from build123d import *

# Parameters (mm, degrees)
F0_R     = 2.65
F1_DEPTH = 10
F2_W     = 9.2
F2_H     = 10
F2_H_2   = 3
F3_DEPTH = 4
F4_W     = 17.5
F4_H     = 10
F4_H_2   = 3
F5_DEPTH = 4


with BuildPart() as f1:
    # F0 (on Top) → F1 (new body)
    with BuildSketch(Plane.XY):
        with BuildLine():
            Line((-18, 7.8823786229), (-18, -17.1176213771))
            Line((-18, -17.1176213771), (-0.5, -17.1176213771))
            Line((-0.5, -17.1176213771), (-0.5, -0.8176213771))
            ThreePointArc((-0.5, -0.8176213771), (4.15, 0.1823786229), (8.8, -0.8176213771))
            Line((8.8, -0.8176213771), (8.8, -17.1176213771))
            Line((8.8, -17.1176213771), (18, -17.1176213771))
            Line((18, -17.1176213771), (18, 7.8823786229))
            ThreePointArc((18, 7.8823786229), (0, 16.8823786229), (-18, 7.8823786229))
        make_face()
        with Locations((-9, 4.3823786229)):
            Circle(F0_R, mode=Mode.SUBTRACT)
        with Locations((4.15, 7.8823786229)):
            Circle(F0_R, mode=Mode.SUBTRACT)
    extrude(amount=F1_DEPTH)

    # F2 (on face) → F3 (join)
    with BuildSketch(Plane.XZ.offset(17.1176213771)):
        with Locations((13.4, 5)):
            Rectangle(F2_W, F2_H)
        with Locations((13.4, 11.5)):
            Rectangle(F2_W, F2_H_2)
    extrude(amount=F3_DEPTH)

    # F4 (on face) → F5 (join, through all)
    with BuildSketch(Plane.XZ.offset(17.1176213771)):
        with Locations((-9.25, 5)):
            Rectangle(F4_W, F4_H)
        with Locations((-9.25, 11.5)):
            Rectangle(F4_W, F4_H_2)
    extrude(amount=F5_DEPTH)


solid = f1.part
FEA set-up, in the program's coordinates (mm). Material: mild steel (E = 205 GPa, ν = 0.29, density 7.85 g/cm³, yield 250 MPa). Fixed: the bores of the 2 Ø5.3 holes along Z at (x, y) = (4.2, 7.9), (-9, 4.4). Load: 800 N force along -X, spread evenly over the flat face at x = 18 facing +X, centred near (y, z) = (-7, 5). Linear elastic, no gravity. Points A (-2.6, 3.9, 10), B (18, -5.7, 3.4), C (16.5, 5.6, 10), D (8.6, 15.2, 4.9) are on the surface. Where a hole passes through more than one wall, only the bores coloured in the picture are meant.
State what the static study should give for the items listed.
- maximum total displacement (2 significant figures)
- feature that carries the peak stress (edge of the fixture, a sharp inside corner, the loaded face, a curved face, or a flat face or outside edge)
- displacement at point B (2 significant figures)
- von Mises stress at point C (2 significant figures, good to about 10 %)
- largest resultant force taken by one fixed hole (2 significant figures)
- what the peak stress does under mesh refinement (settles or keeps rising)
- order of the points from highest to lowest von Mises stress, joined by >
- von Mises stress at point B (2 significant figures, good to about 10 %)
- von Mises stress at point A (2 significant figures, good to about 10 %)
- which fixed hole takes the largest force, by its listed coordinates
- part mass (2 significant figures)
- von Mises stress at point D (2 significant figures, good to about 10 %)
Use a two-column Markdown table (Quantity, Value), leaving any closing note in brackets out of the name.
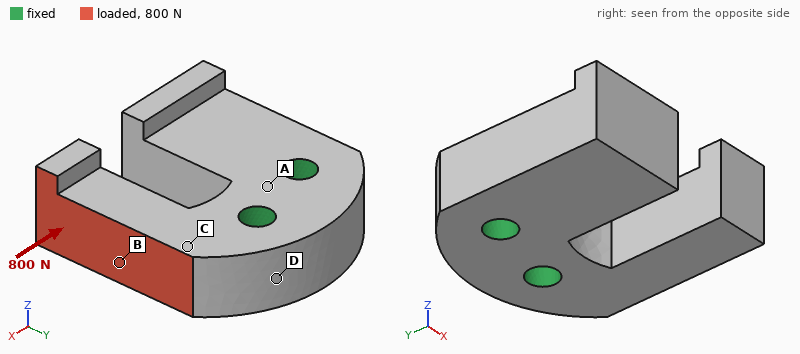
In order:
| Quantity | Value |
|---|---|
| maximum total displacement | 18 µm |
| feature that carries the peak stress | a sharp inside corner |
| displacement at point B | 7.2 µm |
| von Mises stress at point C | 21 MPa |
| largest resultant force taken by one fixed hole | 610 N |
| what the peak stress does under mesh refinement | keeps rising |
| order of the points from highest to lowest von Mises stress, joined by > | B > C > D > A |
| von Mises stress at point B | 27 MPa |
| von Mises stress at point A | 8.5 MPa |
| which fixed hole takes the largest force, by its listed coordinates | (4.2, 7.9) |
| part mass | 83 g |
| von Mises stress at point D | 16 MPa |
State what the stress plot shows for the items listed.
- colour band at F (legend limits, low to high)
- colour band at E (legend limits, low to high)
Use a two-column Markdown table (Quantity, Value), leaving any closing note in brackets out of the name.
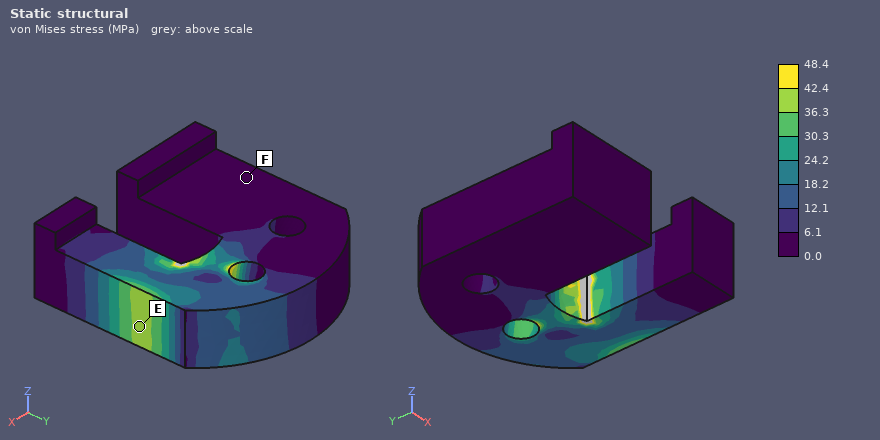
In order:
| Quantity | Value |
|---|---|
| colour band at F | 0.0 to 6.1 MPa |
| colour band at E | 36.3 to 42.4 MPa |
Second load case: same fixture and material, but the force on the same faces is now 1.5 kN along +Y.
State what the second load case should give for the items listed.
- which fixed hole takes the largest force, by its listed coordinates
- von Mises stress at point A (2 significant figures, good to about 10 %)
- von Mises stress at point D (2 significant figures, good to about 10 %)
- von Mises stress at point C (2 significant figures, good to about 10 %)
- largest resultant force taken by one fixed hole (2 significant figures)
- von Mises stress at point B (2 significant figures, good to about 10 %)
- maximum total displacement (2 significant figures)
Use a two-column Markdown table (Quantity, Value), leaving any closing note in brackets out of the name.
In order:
| Quantity | Value |
|---|---|
| which fixed hole takes the largest force, by its listed coordinates | (4.2, 7.9) |
| von Mises stress at point A | 11 MPa |
| von Mises stress at point D | 30 MPa |
| von Mises stress at point C | 32 MPa |
| largest resultant force taken by one fixed hole | 2.1 kN |
| von Mises stress at point B | 37 MPa |
| maximum total displacement | 23 µm |
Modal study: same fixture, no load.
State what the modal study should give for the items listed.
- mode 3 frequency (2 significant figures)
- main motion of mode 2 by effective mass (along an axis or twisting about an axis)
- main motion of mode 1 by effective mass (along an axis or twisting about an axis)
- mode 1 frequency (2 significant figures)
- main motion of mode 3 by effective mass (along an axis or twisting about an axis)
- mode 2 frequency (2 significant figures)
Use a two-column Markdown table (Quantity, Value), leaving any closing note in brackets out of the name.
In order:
| Quantity | Value |
|---|---|
| mode 3 frequency | 11 kHz |
| main motion of mode 2 by effective mass | along X |
| main motion of mode 1 by effective mass | along Z |
| mode 1 frequency | 8000 Hz |
| main motion of mode 3 by effective mass | along Z |
| mode 2 frequency | 8700 Hz |
